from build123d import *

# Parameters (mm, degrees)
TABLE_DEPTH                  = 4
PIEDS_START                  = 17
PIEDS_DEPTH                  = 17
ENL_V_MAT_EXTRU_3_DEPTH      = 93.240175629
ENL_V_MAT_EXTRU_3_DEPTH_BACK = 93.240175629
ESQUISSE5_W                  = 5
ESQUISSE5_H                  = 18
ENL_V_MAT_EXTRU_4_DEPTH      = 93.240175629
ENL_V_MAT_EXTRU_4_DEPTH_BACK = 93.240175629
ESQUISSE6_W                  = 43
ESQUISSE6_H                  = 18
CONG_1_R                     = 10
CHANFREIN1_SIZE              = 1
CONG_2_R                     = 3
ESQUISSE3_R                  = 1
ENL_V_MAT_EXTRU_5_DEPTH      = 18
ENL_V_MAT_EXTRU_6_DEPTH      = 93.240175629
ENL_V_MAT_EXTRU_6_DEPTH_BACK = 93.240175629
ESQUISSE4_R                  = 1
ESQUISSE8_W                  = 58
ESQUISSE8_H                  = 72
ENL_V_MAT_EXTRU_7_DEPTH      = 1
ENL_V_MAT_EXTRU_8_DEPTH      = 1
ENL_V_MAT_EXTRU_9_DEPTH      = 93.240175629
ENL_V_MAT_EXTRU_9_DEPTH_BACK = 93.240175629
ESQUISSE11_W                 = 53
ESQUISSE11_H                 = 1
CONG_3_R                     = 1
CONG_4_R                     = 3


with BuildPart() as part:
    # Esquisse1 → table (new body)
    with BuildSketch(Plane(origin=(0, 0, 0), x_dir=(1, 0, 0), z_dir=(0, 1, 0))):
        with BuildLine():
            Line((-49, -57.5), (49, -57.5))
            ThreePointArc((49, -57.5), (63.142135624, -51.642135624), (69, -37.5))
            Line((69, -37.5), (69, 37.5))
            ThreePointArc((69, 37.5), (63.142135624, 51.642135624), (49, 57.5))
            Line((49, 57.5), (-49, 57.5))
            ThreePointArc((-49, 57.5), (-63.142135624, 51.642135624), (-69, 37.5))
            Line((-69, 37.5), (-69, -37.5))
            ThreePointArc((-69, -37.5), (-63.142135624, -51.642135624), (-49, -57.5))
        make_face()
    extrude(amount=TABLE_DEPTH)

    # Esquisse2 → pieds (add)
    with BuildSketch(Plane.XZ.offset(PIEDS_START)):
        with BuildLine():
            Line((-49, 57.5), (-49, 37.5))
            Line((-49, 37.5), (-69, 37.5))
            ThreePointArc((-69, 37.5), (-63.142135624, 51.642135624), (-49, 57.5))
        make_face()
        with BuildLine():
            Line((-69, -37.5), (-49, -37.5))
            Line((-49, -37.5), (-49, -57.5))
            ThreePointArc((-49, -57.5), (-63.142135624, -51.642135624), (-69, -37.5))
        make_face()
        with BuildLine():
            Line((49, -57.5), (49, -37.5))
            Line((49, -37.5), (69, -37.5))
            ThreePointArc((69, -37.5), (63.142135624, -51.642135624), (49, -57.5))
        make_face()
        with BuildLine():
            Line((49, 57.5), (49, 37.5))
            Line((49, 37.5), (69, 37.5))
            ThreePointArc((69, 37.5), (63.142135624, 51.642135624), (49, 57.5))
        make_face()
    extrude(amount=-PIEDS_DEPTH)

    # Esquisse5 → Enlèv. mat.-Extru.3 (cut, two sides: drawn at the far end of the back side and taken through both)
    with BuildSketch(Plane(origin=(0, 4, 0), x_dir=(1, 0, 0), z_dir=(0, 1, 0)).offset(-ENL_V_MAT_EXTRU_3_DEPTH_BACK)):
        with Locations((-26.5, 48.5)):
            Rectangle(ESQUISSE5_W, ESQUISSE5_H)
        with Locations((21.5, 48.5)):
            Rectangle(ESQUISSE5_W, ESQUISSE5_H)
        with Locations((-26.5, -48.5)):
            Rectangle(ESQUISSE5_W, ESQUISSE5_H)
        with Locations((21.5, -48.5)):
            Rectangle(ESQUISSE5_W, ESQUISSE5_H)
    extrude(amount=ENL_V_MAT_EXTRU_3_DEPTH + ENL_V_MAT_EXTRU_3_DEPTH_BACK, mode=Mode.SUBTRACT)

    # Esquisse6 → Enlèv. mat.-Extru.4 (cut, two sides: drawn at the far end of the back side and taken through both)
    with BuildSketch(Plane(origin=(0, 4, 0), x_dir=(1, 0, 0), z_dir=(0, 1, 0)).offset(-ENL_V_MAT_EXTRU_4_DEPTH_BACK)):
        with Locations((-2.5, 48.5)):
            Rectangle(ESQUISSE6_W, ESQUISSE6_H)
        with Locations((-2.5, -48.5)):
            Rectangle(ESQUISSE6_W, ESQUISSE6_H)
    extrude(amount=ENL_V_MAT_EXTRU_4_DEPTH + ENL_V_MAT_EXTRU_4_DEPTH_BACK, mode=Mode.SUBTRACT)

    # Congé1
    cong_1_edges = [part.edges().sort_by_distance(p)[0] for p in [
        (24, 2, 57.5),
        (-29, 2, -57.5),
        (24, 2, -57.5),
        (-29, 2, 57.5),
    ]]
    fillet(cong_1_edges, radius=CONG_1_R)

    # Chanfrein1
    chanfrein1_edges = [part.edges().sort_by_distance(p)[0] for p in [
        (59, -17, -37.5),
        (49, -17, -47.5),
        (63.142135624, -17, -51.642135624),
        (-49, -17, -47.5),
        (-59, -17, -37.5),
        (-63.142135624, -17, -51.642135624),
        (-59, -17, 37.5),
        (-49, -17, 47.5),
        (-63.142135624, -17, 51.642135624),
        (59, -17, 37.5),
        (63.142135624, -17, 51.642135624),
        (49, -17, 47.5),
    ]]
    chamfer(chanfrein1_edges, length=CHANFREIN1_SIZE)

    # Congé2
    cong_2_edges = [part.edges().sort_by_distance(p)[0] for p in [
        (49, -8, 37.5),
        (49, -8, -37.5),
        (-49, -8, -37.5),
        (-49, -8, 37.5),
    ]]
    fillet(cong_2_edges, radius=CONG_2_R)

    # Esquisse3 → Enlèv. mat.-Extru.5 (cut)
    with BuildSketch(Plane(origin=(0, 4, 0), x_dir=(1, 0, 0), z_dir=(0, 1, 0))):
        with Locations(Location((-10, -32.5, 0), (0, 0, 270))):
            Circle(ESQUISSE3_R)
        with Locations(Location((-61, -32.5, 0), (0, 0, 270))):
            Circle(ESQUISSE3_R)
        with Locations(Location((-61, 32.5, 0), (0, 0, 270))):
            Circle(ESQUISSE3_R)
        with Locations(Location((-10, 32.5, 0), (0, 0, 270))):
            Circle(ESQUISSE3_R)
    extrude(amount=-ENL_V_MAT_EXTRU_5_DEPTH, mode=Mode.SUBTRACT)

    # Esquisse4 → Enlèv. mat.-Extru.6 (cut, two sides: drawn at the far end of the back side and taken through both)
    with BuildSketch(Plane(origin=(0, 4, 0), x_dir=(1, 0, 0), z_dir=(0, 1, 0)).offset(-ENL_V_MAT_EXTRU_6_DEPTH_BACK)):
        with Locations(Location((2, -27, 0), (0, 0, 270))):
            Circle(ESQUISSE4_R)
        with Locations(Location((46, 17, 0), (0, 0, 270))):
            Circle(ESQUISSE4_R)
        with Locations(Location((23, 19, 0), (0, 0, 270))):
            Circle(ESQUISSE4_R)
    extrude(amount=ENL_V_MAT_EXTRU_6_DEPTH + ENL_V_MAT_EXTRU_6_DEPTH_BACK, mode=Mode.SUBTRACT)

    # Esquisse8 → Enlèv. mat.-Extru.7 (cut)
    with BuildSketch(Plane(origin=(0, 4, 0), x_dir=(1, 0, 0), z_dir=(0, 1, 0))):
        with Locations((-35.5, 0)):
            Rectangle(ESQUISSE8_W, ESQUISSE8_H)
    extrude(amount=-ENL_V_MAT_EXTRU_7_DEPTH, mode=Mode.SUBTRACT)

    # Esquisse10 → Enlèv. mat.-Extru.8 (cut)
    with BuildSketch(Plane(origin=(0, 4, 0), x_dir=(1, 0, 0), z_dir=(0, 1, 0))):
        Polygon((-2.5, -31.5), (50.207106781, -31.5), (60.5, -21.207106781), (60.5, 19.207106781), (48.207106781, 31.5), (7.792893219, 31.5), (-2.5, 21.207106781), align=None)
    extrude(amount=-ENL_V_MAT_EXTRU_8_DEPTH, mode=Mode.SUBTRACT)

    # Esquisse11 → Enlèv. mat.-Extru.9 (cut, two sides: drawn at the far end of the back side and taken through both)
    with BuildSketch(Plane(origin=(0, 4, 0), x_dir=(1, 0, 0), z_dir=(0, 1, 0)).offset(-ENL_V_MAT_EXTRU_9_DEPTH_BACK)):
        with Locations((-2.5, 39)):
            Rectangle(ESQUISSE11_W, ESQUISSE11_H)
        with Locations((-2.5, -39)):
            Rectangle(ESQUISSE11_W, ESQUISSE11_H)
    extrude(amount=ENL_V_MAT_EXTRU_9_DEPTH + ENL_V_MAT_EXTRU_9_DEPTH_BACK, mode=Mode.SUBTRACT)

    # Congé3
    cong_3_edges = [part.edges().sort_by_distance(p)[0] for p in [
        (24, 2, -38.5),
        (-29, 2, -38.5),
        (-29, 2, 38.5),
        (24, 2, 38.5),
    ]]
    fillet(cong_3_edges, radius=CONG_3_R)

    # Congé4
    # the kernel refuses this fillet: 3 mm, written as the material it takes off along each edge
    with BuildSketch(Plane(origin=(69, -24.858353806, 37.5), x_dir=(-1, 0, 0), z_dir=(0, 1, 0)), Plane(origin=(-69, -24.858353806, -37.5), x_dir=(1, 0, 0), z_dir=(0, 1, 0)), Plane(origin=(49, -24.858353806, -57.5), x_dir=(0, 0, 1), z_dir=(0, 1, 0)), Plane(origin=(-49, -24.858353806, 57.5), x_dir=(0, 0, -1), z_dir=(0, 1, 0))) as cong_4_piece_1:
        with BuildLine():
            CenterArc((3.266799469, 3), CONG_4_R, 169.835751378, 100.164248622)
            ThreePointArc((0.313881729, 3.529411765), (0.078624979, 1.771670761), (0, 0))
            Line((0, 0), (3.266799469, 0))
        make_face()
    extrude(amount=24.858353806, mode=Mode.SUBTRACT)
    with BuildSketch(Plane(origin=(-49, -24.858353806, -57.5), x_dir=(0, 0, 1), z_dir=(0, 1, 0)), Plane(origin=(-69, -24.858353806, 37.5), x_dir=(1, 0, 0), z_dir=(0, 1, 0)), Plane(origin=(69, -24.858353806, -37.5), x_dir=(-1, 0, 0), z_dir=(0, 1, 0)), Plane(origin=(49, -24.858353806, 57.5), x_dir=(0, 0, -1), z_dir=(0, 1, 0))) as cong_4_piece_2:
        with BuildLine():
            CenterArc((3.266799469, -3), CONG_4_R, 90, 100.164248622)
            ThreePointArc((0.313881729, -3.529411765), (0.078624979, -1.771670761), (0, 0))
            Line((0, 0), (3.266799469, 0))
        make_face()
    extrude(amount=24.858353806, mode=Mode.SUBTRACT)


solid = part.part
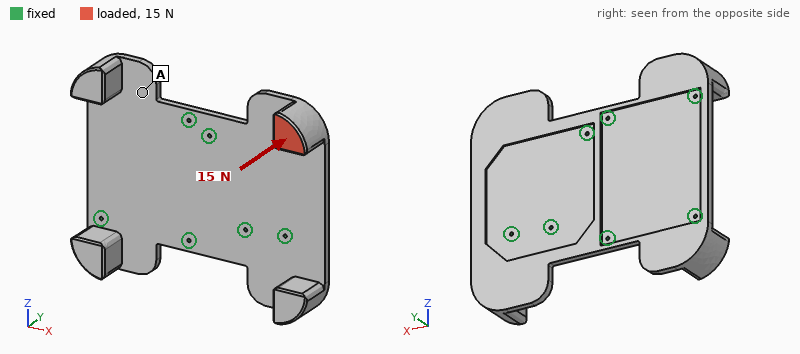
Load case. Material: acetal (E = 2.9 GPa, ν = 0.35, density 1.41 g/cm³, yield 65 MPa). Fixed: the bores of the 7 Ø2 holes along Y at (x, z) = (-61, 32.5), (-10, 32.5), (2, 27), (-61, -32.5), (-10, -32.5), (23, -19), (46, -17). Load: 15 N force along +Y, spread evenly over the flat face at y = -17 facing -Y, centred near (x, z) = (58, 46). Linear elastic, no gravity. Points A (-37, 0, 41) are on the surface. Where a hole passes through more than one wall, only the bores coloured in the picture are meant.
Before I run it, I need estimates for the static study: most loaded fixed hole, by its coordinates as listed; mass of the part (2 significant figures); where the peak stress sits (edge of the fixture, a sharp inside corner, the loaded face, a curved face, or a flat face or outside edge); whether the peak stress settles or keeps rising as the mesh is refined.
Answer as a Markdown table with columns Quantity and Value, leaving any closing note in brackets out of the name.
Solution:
| Quantity | Value |
|---|---|
| most loaded fixed hole, by its coordinates as listed | (2, 27) |
| mass of the part | 94 g |
| where the peak stress sits | edge of the fixture |
| whether the peak stress settles or keeps rising as the mesh is refined | keeps rising |
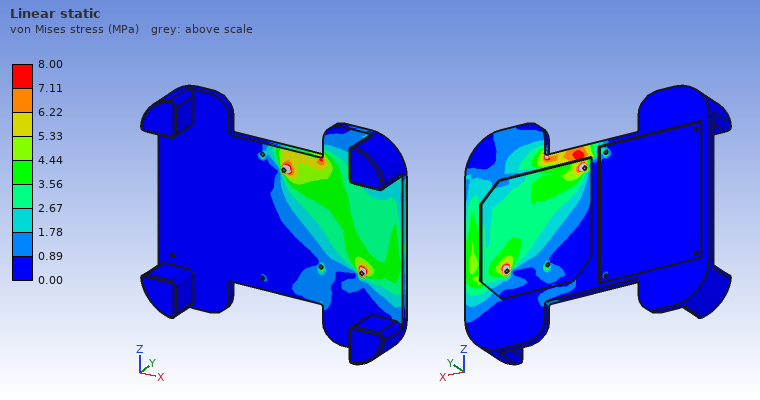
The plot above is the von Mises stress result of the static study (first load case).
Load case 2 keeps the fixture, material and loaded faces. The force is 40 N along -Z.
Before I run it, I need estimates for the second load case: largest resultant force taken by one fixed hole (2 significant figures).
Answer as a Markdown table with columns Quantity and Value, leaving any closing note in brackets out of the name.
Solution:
| Quantity | Value |
|---|---|
| largest resultant force taken by one fixed hole | 25 N |
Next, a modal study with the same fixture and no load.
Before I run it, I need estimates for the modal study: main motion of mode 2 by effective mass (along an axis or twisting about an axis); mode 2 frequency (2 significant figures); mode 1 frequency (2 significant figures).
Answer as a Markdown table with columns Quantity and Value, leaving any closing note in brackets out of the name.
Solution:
| Quantity | Value |
|---|---|
| main motion of mode 2 by effective mass | along Y |
| mode 2 frequency | 260 Hz |
| mode 1 frequency | 140 Hz |
